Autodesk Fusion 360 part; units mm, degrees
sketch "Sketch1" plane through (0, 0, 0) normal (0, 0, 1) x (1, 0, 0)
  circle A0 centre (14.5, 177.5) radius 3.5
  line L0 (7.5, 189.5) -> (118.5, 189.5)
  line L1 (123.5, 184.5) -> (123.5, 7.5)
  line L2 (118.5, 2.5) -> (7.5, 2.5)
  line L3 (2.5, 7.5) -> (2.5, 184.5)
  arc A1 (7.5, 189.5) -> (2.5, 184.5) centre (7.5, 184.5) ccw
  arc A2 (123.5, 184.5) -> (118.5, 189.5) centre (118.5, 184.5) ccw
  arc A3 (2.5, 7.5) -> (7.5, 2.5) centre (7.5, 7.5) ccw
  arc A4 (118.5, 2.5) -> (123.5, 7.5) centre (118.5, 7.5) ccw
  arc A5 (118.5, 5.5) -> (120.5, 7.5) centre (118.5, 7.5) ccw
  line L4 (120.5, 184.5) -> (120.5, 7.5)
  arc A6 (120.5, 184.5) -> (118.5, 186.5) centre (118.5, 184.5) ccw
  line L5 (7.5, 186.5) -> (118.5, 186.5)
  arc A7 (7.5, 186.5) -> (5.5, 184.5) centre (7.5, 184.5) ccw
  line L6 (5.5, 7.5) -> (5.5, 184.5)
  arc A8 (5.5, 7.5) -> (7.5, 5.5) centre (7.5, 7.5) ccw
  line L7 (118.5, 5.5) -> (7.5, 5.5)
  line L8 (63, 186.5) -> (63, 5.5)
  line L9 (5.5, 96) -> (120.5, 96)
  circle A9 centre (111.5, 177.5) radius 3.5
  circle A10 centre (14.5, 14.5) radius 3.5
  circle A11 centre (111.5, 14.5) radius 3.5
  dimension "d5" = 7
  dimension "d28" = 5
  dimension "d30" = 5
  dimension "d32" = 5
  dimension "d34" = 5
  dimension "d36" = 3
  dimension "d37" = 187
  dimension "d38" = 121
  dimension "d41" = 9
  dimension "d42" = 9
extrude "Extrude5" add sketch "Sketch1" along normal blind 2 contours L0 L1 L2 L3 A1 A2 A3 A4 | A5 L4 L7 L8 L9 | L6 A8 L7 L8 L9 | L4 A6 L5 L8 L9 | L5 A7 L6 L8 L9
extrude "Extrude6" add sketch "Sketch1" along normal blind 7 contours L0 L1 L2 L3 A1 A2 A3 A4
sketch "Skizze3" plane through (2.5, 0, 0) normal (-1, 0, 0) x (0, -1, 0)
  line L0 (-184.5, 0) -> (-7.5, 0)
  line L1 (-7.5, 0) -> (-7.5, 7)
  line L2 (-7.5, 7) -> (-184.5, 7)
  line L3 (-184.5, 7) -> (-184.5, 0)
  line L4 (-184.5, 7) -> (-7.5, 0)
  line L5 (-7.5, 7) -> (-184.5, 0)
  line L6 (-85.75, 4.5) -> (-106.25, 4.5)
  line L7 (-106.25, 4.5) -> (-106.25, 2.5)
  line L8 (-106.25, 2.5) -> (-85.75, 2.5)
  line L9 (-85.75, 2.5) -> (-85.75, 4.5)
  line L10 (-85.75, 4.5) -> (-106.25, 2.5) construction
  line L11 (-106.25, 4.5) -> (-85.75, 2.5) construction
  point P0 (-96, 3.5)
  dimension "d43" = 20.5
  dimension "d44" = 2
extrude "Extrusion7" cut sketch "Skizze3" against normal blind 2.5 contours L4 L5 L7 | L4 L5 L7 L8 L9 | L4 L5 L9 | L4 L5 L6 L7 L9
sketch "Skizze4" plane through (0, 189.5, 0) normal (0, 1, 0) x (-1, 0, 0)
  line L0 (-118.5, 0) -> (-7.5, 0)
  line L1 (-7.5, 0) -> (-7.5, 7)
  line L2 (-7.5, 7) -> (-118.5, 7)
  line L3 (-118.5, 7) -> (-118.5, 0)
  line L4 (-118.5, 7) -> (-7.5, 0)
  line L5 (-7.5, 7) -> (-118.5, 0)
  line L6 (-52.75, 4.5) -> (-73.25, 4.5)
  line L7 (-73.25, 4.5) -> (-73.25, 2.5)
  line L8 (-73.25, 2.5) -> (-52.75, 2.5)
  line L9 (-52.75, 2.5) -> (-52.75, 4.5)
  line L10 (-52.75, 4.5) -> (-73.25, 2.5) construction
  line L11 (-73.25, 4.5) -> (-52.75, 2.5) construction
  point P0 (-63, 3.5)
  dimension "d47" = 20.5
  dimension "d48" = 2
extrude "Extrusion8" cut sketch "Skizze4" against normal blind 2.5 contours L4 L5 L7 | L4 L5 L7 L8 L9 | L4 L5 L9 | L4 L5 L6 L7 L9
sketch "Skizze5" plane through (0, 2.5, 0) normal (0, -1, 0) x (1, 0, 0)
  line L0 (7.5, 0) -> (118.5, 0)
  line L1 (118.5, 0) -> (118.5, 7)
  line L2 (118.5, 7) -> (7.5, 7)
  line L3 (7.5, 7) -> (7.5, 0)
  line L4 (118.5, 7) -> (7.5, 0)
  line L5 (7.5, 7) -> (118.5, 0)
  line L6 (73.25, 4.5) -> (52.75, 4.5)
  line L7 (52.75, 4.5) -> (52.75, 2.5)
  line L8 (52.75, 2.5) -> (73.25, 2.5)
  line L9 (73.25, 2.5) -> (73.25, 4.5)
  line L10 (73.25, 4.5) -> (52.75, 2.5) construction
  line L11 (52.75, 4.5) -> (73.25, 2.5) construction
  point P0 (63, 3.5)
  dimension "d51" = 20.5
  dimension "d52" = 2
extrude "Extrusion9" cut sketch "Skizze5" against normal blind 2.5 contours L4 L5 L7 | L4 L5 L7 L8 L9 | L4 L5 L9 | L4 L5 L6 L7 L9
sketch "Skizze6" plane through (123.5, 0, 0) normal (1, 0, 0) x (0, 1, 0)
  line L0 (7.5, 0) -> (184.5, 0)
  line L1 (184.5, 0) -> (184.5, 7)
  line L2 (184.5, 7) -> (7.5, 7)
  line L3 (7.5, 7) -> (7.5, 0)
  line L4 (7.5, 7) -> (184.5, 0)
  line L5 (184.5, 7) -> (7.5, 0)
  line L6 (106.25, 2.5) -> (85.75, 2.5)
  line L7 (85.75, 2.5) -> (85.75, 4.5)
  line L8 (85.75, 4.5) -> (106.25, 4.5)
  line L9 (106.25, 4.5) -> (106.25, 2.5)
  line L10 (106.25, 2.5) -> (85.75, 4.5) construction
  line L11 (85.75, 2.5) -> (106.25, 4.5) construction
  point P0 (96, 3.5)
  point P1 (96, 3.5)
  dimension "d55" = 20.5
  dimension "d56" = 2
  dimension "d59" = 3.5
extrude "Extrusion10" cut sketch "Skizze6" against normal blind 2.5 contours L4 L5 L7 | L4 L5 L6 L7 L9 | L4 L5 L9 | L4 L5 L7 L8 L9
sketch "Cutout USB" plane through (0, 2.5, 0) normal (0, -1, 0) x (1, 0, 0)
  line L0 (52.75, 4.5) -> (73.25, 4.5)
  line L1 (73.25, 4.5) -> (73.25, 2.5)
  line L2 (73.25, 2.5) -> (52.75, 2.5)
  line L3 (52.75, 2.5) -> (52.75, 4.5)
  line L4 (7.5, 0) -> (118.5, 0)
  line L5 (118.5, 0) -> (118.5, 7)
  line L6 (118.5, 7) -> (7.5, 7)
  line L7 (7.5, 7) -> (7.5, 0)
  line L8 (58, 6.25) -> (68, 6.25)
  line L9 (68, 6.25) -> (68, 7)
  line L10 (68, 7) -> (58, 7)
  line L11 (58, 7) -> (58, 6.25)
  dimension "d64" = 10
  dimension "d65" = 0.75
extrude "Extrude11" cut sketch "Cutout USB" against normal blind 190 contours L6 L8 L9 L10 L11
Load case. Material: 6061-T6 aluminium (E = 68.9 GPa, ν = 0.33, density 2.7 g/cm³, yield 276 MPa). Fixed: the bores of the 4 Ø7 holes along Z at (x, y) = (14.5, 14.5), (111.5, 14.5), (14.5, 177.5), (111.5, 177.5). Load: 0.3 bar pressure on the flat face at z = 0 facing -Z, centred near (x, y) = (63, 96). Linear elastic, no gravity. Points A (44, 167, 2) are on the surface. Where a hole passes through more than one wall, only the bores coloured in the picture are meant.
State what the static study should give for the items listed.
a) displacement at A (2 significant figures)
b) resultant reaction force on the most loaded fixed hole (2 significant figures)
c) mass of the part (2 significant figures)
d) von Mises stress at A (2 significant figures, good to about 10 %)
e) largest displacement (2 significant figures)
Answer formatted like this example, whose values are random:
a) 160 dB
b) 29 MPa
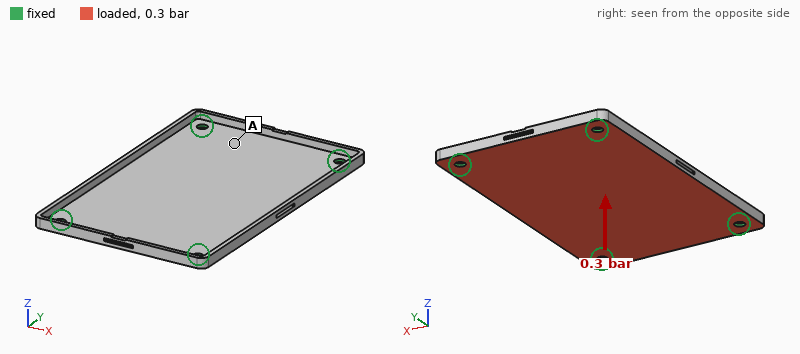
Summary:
a) 0.19 mm
b) 190 N
c) 140 g
d) 19 MPa
e) 0.79 mm
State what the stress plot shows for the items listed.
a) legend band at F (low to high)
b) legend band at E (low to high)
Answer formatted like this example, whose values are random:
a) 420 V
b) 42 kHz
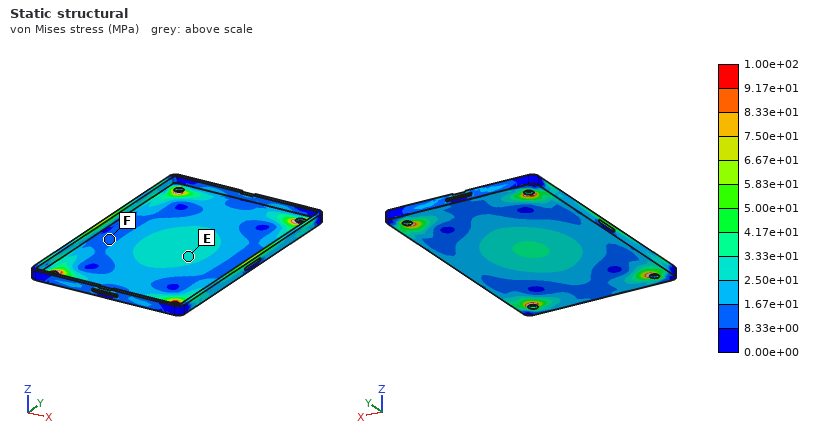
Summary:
a) 8.33e+00 to 1.67e+01 MPa
b) 2.50e+01 to 3.33e+01 MPa
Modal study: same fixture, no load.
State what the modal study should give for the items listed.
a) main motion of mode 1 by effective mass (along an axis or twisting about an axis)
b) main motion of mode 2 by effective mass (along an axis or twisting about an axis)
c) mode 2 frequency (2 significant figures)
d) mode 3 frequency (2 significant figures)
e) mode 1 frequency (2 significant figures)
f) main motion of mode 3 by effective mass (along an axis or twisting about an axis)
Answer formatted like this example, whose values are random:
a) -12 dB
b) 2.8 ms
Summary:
a) along Z
b) twisting about Y
c) 880 Hz
d) 1100 Hz
e) 520 Hz
f) twisting about X
